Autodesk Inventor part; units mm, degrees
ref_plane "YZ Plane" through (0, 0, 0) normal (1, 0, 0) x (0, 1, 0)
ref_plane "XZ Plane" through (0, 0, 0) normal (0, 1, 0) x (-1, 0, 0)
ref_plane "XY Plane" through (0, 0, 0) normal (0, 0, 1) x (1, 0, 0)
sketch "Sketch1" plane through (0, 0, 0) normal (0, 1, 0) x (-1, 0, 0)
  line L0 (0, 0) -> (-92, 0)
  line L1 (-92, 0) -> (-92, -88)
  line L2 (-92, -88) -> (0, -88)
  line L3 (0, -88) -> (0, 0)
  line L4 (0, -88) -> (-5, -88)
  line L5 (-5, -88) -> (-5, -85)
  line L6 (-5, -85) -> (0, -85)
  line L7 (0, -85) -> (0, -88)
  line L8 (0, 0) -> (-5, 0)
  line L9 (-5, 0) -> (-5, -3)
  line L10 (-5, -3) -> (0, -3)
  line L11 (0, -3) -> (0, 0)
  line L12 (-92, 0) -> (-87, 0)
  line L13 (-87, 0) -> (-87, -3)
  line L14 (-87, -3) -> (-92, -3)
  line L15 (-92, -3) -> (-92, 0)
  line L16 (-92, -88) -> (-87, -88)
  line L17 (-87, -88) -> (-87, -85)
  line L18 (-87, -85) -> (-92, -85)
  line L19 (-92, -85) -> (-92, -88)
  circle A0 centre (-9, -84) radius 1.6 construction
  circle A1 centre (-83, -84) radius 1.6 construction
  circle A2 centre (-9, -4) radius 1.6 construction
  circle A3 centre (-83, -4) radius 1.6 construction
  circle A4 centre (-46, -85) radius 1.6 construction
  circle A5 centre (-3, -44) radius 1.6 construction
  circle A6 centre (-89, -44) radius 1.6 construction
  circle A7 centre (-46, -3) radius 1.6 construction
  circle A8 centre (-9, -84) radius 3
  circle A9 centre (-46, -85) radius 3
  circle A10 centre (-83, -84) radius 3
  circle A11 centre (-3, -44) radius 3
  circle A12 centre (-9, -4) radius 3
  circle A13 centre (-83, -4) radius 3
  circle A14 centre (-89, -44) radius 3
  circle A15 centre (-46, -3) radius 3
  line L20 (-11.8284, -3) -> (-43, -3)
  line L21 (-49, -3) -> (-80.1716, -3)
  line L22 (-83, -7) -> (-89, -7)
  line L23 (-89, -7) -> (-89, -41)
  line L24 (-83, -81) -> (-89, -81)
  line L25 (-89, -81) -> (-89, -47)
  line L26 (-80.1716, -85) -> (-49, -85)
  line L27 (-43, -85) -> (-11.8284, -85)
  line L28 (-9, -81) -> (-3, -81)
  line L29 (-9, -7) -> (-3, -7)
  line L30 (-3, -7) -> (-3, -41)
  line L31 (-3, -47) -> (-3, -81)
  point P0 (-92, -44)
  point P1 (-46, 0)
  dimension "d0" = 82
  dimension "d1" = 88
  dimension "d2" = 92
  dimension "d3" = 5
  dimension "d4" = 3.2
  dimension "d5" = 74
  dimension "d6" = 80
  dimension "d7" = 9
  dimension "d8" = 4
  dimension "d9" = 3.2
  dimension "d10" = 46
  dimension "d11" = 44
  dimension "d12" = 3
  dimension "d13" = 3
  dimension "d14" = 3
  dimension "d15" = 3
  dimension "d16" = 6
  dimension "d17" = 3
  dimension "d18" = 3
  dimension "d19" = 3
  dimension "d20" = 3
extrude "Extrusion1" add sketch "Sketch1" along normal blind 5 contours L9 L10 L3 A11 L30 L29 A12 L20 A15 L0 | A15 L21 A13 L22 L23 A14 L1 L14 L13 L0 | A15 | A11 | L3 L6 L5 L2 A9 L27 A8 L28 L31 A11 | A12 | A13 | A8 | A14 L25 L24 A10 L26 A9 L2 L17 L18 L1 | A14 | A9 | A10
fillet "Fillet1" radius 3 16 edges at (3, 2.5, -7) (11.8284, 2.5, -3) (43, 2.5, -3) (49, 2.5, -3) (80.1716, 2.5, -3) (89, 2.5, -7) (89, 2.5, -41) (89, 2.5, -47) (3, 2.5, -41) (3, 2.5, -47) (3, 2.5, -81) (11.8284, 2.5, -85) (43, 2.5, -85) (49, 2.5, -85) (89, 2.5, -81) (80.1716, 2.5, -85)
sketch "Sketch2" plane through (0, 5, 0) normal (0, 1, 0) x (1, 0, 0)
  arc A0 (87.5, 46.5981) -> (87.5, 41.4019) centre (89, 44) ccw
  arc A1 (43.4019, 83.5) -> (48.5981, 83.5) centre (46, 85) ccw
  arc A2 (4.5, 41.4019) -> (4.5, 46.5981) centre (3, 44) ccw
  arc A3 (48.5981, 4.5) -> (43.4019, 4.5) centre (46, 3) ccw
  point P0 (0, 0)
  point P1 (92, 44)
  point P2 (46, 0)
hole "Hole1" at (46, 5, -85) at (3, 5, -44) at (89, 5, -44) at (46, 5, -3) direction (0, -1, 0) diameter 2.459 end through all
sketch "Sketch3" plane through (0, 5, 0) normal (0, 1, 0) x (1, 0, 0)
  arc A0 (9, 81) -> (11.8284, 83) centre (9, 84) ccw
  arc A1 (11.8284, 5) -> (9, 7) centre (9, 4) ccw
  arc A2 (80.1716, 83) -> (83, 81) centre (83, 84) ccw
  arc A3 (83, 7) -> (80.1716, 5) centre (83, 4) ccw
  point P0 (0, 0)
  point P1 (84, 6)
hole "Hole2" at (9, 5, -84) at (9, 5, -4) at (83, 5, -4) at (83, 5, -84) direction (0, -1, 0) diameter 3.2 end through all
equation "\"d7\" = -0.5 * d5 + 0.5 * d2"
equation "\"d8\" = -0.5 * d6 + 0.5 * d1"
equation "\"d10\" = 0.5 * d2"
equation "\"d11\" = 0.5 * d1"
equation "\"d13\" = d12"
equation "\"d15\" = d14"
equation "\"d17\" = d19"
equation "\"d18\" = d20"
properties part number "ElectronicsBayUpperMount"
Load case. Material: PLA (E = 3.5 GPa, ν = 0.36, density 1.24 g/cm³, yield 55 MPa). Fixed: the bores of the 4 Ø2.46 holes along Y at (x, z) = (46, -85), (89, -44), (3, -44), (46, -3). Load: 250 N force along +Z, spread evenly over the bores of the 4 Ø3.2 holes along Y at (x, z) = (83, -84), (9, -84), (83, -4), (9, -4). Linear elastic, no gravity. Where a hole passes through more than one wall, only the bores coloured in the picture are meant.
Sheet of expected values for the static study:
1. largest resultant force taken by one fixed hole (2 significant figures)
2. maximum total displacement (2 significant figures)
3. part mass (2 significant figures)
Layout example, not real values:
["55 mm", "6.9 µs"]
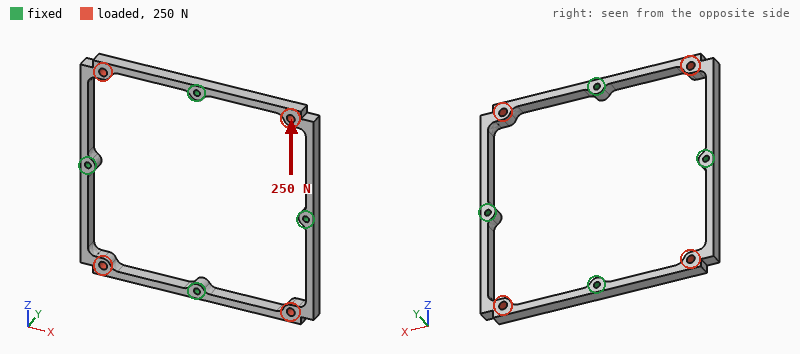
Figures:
["110 N", "0.38 mm", "7.1 g"]
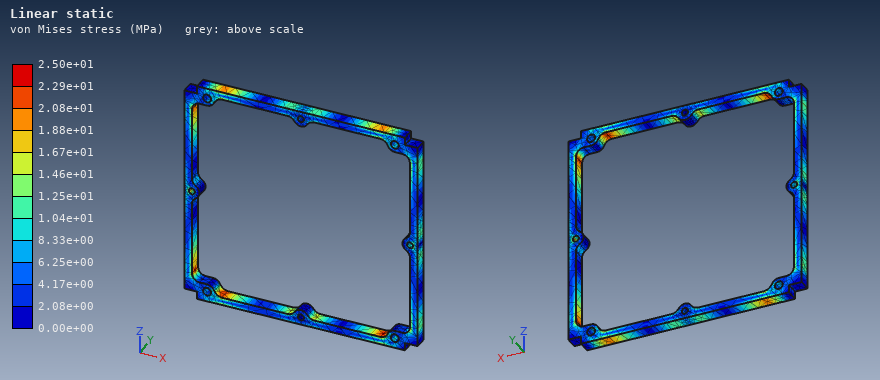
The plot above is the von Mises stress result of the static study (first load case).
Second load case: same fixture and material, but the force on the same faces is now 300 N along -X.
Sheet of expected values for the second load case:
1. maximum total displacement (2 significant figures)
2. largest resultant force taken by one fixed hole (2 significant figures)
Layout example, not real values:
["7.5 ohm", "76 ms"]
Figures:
["0.15 mm", "140 N"]
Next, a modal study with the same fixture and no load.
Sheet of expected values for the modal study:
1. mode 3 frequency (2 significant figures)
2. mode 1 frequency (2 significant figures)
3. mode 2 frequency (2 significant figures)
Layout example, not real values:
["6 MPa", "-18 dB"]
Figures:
["820 Hz", "820 Hz", "820 Hz"]
